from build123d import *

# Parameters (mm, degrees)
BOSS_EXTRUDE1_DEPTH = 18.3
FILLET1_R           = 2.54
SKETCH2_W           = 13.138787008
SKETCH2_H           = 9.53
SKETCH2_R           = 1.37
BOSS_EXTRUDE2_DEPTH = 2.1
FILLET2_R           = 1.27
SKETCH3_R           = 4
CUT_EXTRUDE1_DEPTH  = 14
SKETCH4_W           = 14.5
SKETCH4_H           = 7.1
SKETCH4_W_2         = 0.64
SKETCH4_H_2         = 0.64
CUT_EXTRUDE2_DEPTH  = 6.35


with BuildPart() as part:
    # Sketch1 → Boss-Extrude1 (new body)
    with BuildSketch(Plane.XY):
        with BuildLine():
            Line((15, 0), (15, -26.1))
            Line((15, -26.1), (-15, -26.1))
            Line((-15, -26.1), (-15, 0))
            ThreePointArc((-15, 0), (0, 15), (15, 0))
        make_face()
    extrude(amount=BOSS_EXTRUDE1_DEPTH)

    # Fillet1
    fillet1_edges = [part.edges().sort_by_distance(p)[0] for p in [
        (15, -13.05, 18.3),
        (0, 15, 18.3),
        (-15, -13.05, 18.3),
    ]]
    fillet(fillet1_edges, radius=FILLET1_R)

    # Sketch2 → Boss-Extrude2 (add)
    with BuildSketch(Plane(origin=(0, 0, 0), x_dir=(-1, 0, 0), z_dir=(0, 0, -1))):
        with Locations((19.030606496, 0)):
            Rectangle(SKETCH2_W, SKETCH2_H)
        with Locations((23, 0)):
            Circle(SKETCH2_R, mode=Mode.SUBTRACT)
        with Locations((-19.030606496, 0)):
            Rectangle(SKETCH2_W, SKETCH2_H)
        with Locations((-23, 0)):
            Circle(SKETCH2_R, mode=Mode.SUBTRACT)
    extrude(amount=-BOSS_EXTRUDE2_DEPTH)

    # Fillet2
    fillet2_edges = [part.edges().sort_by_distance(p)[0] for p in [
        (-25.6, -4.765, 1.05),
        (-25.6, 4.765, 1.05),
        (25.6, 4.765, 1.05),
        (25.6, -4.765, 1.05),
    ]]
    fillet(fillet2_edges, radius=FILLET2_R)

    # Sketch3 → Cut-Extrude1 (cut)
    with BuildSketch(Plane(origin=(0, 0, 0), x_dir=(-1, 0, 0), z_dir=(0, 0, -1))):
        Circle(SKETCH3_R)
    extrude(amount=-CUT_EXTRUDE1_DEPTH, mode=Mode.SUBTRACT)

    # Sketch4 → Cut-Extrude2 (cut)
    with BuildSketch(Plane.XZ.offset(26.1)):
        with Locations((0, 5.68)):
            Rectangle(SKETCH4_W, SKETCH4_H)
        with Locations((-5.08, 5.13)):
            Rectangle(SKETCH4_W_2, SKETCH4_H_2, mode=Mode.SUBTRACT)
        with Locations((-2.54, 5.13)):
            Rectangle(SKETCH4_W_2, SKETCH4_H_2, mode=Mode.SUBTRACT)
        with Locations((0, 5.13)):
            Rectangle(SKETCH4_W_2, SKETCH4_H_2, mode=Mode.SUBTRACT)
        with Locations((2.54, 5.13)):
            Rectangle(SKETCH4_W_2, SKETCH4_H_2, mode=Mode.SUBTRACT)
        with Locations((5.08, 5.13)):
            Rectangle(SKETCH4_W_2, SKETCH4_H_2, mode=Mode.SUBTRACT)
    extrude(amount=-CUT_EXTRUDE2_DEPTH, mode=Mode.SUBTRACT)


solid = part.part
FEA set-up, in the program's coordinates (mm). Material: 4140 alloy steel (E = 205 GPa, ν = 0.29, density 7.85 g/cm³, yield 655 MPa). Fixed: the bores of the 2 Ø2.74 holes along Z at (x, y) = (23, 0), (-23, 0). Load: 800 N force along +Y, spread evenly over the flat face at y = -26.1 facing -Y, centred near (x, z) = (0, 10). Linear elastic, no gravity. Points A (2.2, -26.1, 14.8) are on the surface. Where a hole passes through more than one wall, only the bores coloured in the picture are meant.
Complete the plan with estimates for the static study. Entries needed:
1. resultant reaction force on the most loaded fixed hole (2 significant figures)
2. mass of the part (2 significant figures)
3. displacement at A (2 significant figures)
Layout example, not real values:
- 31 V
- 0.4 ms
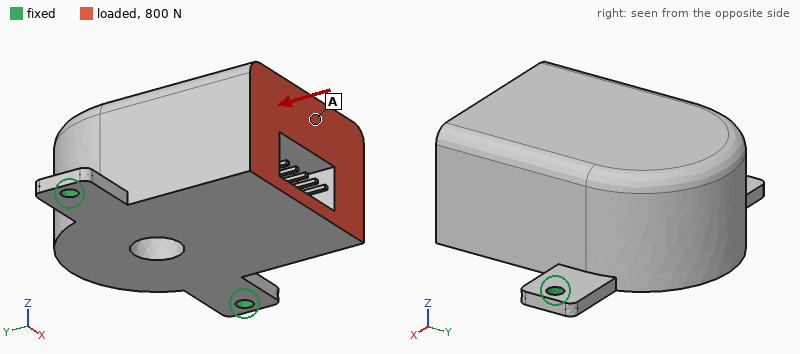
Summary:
- 400 N
- 150 g
- 0.33 mm
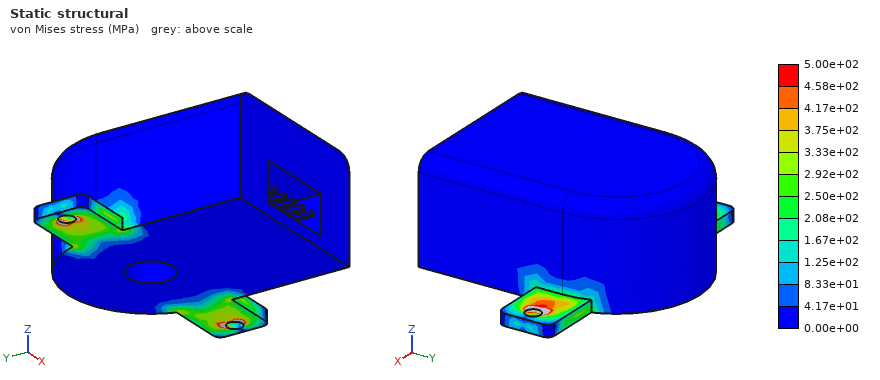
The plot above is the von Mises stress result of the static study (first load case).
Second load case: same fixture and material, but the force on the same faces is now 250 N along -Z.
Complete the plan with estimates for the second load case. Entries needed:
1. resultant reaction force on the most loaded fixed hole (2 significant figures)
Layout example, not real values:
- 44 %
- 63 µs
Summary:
- 140 N
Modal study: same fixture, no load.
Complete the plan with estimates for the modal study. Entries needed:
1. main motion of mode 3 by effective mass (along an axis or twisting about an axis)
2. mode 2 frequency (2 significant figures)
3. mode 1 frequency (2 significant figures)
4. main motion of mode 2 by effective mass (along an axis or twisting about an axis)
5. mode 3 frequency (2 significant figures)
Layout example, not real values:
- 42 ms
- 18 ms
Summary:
- along X
- 3100 Hz
- 630 Hz
- along Z
- 3900 Hz
